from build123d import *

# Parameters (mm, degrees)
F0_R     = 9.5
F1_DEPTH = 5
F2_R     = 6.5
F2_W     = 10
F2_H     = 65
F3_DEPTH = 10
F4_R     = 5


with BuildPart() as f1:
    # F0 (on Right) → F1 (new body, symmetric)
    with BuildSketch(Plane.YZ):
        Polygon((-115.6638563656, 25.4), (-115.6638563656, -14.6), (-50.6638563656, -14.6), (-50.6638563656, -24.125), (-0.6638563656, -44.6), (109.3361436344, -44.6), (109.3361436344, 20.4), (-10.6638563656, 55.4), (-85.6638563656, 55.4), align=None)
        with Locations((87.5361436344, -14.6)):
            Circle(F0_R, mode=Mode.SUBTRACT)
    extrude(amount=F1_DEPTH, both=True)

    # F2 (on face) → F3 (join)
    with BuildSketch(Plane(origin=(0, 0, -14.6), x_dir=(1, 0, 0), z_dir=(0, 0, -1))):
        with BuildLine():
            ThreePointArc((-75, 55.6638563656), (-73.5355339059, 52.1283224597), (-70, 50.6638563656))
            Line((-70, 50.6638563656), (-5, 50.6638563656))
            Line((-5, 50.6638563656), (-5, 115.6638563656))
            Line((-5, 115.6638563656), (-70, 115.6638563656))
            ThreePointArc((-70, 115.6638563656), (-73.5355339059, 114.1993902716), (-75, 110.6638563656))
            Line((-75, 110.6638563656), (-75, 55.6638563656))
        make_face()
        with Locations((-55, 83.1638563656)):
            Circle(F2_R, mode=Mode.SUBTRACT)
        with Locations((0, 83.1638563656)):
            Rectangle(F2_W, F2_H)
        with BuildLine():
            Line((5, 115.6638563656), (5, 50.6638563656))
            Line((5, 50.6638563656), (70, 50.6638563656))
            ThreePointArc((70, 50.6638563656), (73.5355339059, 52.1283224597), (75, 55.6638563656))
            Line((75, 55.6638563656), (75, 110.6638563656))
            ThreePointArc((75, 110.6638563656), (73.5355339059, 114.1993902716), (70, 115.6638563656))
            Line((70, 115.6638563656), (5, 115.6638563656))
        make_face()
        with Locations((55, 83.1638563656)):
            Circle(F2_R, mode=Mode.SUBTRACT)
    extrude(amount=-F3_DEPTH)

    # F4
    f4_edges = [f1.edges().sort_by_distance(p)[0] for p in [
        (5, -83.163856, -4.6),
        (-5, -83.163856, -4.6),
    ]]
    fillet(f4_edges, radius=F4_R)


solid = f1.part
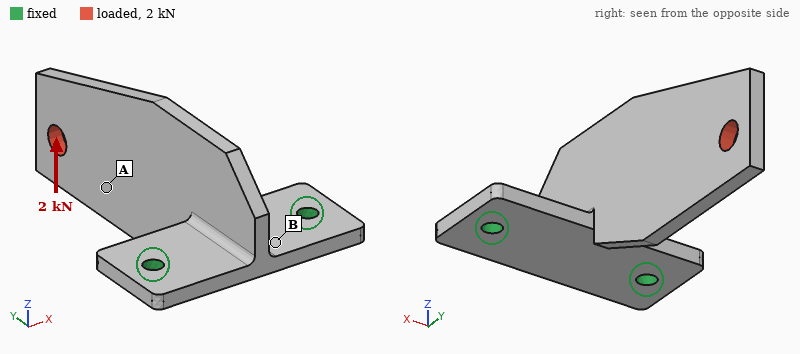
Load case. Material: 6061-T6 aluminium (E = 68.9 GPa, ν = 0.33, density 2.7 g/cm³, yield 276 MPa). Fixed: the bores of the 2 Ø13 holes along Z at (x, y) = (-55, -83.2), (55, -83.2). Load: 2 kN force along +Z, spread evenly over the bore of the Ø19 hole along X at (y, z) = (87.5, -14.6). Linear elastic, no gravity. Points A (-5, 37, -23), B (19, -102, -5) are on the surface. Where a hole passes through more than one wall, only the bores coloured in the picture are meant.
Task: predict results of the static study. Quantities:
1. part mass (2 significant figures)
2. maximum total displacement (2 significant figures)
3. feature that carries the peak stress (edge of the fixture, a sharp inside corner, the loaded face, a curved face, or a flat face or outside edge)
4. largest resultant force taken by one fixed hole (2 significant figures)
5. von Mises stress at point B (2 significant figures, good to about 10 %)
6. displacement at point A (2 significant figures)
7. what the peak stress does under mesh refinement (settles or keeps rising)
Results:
700 g
2.6 mm
edge of the fixture
1.2 kN
89 MPa
1.6 mm
keeps rising
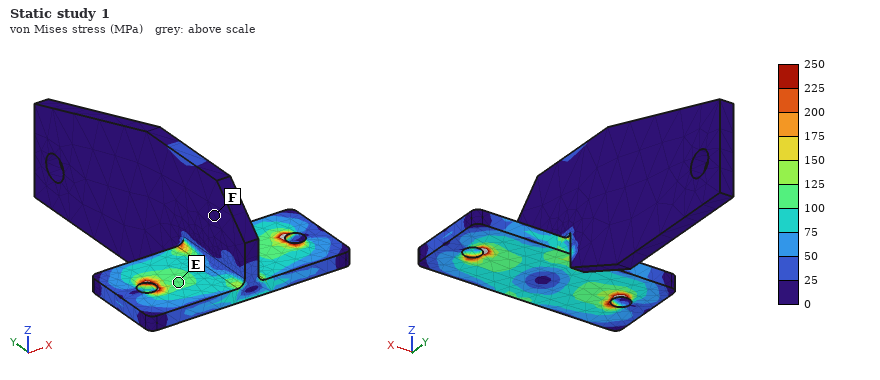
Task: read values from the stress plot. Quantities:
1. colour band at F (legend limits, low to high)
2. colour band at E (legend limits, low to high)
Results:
0 to 25 MPa
100 to 125 MPa
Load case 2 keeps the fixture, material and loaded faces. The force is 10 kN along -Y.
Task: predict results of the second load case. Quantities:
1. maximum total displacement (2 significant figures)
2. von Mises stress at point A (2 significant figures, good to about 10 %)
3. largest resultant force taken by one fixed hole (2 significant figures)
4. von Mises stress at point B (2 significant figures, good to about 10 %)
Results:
0.51 mm
17 MPa
5.1 kN
16 MPa
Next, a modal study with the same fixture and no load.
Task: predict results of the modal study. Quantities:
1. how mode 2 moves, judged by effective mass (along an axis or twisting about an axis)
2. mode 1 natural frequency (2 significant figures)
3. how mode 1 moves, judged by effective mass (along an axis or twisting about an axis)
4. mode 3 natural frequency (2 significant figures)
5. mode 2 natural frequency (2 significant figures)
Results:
along Z
280 Hz
along X
900 Hz
350 Hz
